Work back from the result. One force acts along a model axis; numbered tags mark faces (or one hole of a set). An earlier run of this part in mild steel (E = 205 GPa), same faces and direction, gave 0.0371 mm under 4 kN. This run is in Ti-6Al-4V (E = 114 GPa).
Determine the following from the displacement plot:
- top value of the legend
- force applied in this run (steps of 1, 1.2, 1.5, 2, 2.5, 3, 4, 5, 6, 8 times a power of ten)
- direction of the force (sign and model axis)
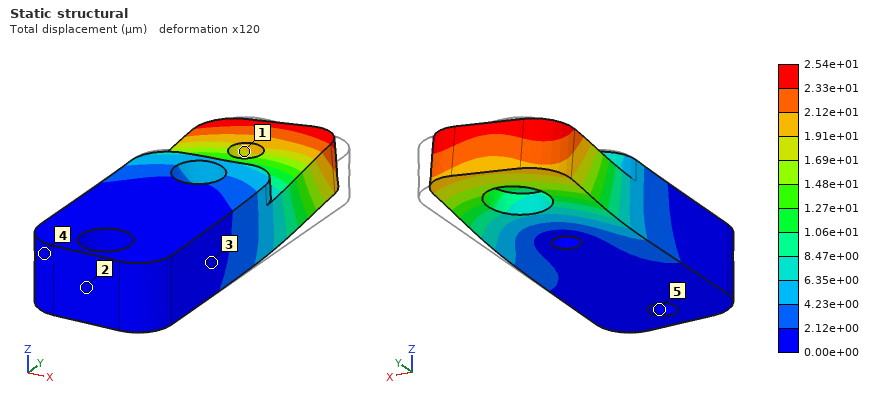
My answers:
2.54e+01 µm
1.5 kN
-X
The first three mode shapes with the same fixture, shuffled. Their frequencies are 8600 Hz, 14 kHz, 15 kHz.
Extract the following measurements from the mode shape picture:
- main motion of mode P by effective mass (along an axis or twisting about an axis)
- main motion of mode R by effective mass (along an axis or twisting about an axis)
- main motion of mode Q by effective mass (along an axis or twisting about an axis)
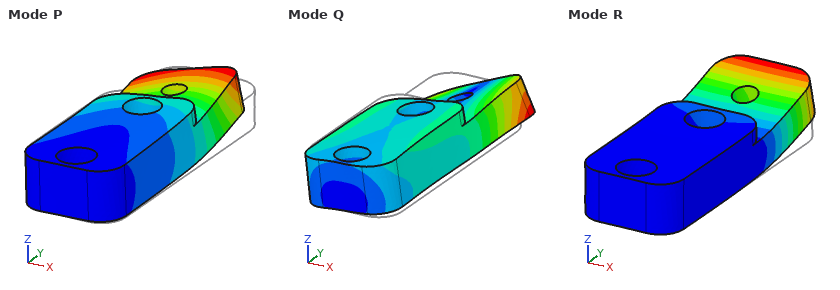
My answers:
along X
along Z
twisting about Y
